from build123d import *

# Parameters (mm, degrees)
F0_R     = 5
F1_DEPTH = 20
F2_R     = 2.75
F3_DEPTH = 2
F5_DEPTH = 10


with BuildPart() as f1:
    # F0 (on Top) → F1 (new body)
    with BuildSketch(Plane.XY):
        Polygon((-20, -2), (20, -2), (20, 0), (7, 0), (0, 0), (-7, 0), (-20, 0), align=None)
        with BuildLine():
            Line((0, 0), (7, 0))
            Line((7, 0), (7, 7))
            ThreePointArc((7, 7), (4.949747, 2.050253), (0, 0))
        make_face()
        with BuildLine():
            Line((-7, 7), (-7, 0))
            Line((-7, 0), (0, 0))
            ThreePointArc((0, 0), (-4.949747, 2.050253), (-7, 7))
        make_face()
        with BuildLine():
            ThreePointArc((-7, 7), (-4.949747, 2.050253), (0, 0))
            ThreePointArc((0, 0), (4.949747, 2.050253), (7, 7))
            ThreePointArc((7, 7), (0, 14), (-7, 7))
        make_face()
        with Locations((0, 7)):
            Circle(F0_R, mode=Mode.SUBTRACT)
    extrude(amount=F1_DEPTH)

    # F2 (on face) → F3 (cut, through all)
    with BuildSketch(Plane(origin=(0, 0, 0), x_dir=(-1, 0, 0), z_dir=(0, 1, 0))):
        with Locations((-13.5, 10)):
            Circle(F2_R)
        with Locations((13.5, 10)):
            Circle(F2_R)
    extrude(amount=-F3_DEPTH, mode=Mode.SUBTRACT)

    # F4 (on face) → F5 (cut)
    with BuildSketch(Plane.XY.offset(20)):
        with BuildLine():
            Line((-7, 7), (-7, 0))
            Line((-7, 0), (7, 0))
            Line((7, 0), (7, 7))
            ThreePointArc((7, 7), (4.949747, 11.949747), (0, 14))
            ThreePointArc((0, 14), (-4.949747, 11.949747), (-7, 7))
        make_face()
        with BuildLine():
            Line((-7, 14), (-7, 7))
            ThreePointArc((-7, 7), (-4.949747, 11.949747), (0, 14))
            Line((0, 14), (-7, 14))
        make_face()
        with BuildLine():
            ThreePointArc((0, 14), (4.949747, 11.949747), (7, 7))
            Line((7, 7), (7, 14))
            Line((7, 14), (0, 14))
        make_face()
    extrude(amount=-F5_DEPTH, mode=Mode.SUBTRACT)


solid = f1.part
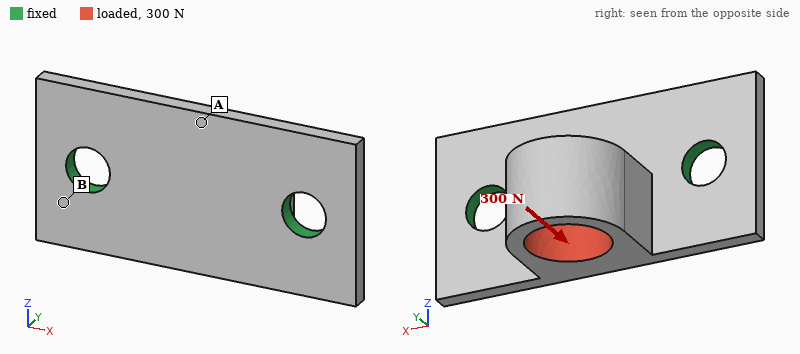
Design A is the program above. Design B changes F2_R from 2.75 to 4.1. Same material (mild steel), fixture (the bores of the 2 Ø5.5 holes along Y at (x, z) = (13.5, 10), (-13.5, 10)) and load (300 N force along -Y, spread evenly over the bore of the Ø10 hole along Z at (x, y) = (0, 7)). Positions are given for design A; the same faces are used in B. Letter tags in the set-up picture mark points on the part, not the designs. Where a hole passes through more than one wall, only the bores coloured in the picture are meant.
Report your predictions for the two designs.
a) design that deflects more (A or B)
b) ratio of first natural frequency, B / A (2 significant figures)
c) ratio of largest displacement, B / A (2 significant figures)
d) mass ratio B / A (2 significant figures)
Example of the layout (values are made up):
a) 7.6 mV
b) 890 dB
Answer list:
a) A
b) 1.3
c) 0.60
d) 0.95
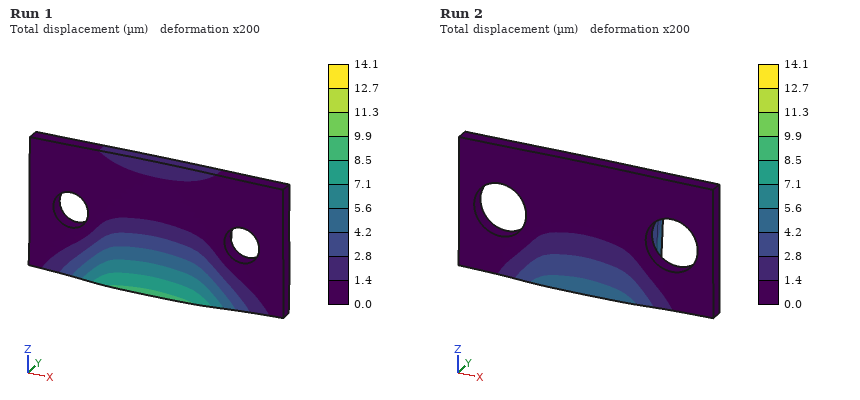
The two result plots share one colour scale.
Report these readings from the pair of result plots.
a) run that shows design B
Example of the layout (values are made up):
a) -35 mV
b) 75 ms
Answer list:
a) Run 2
